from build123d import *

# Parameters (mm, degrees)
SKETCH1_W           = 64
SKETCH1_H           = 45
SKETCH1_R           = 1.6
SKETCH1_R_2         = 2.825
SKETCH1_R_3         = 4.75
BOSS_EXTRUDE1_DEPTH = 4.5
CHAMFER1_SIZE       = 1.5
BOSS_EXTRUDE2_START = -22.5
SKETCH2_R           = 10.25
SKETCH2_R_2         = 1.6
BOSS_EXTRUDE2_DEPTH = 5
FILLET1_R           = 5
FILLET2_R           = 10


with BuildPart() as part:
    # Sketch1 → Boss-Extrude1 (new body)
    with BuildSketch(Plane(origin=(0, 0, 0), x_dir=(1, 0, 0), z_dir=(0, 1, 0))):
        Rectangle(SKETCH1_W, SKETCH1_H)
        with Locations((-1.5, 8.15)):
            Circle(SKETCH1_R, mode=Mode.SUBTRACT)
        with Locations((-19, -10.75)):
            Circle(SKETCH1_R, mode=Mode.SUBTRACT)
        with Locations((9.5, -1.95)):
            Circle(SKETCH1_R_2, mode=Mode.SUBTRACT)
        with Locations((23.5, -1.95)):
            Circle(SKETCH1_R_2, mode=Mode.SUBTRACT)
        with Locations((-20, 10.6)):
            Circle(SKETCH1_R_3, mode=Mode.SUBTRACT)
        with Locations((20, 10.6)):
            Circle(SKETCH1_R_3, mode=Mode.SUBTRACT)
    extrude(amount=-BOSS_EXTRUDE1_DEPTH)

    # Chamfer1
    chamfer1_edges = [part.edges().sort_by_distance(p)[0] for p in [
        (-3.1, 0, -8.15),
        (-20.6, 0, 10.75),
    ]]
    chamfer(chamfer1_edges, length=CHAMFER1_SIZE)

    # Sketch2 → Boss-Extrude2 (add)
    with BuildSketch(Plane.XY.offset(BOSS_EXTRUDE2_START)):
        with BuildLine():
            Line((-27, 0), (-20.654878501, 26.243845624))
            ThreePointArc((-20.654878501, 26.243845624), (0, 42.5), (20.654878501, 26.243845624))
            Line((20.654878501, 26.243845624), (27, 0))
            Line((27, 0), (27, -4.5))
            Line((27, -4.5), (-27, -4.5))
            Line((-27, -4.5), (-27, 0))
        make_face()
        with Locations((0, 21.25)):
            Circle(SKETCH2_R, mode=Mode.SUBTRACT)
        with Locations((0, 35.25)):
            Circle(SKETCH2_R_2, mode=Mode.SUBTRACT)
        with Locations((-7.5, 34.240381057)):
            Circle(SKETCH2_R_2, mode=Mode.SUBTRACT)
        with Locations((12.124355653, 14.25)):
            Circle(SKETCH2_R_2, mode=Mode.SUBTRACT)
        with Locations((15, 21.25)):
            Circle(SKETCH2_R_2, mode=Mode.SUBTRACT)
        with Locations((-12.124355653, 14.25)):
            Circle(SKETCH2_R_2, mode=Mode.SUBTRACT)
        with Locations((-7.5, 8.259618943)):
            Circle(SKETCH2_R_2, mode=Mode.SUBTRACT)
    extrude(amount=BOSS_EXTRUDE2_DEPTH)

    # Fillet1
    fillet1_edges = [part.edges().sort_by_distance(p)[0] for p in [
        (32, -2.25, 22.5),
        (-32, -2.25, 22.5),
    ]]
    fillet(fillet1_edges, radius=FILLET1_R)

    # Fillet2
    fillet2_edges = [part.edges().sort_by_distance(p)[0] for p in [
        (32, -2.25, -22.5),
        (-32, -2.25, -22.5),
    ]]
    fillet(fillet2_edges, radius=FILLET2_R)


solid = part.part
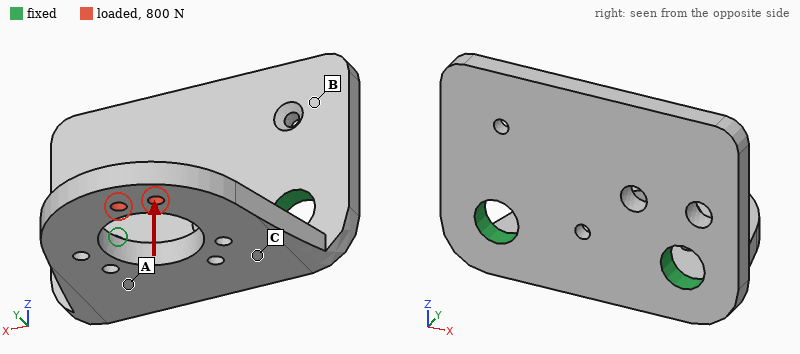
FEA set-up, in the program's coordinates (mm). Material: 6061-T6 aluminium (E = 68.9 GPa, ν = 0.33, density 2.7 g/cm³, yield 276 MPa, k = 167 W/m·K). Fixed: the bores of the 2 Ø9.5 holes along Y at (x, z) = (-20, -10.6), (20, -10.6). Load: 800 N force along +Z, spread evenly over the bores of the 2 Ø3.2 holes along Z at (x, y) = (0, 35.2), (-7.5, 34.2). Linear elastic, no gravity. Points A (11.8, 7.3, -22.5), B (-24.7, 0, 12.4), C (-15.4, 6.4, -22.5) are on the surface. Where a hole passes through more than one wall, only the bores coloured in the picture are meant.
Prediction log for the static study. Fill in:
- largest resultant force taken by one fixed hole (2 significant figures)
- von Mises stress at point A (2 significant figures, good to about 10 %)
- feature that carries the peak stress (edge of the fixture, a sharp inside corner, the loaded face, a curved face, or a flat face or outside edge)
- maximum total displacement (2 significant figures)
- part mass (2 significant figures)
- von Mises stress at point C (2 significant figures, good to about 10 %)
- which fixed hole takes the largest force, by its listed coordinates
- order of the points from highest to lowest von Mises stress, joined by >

480 N
92 MPa
a curved face
0.98 mm
50 g
130 MPa
(-20, -10.6)
C > A > B
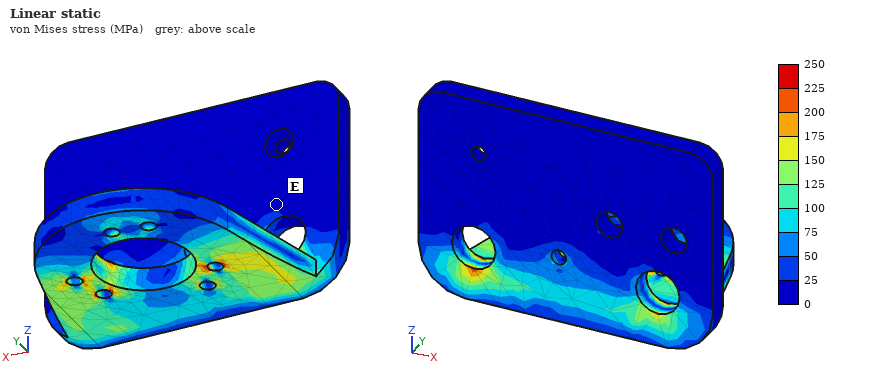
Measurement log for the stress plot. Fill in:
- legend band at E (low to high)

0 to 25 MPa
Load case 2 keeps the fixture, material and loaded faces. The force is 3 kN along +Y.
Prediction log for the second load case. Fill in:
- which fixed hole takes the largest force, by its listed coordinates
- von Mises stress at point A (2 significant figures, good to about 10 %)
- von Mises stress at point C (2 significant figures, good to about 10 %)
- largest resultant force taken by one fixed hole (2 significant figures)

(-20, -10.6)
12 MPa
22 MPa
1.8 kN
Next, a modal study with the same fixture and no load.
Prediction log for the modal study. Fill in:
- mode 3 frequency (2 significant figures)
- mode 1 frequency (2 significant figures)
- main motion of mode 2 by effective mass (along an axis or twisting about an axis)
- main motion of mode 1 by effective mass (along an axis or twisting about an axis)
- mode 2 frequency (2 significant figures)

5600 Hz
2100 Hz
along Y
along Z
3700 Hz
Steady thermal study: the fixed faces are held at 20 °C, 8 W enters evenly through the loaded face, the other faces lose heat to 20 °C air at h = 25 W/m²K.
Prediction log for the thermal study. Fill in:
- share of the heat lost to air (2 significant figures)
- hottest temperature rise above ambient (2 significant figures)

9.2 %
17 K
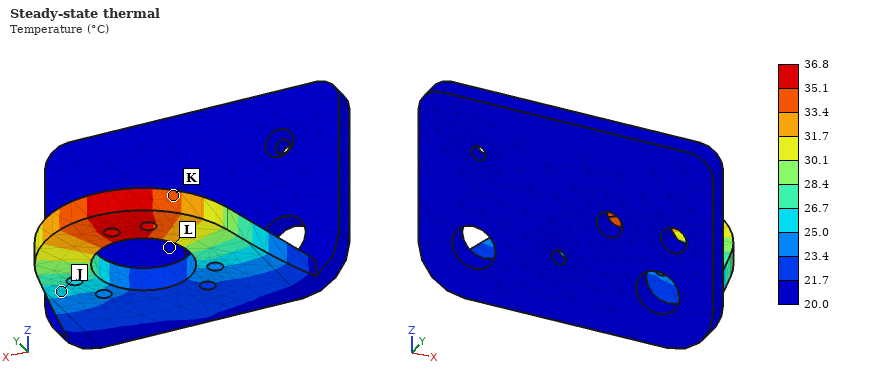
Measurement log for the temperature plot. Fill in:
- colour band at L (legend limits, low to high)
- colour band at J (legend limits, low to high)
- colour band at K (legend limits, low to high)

20.0 to 21.7 °C
25.0 to 26.7 °C
33.4 to 35.1 °C
